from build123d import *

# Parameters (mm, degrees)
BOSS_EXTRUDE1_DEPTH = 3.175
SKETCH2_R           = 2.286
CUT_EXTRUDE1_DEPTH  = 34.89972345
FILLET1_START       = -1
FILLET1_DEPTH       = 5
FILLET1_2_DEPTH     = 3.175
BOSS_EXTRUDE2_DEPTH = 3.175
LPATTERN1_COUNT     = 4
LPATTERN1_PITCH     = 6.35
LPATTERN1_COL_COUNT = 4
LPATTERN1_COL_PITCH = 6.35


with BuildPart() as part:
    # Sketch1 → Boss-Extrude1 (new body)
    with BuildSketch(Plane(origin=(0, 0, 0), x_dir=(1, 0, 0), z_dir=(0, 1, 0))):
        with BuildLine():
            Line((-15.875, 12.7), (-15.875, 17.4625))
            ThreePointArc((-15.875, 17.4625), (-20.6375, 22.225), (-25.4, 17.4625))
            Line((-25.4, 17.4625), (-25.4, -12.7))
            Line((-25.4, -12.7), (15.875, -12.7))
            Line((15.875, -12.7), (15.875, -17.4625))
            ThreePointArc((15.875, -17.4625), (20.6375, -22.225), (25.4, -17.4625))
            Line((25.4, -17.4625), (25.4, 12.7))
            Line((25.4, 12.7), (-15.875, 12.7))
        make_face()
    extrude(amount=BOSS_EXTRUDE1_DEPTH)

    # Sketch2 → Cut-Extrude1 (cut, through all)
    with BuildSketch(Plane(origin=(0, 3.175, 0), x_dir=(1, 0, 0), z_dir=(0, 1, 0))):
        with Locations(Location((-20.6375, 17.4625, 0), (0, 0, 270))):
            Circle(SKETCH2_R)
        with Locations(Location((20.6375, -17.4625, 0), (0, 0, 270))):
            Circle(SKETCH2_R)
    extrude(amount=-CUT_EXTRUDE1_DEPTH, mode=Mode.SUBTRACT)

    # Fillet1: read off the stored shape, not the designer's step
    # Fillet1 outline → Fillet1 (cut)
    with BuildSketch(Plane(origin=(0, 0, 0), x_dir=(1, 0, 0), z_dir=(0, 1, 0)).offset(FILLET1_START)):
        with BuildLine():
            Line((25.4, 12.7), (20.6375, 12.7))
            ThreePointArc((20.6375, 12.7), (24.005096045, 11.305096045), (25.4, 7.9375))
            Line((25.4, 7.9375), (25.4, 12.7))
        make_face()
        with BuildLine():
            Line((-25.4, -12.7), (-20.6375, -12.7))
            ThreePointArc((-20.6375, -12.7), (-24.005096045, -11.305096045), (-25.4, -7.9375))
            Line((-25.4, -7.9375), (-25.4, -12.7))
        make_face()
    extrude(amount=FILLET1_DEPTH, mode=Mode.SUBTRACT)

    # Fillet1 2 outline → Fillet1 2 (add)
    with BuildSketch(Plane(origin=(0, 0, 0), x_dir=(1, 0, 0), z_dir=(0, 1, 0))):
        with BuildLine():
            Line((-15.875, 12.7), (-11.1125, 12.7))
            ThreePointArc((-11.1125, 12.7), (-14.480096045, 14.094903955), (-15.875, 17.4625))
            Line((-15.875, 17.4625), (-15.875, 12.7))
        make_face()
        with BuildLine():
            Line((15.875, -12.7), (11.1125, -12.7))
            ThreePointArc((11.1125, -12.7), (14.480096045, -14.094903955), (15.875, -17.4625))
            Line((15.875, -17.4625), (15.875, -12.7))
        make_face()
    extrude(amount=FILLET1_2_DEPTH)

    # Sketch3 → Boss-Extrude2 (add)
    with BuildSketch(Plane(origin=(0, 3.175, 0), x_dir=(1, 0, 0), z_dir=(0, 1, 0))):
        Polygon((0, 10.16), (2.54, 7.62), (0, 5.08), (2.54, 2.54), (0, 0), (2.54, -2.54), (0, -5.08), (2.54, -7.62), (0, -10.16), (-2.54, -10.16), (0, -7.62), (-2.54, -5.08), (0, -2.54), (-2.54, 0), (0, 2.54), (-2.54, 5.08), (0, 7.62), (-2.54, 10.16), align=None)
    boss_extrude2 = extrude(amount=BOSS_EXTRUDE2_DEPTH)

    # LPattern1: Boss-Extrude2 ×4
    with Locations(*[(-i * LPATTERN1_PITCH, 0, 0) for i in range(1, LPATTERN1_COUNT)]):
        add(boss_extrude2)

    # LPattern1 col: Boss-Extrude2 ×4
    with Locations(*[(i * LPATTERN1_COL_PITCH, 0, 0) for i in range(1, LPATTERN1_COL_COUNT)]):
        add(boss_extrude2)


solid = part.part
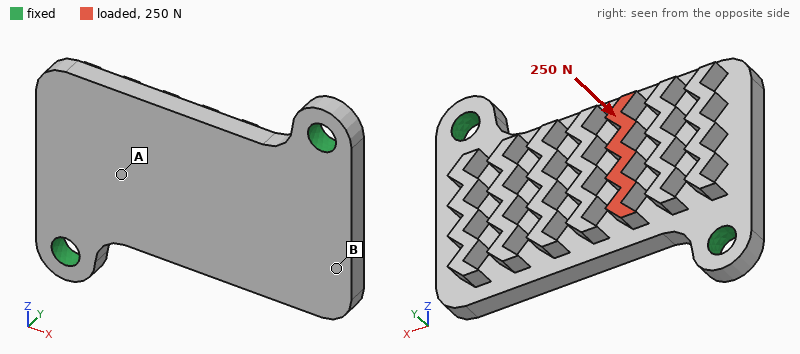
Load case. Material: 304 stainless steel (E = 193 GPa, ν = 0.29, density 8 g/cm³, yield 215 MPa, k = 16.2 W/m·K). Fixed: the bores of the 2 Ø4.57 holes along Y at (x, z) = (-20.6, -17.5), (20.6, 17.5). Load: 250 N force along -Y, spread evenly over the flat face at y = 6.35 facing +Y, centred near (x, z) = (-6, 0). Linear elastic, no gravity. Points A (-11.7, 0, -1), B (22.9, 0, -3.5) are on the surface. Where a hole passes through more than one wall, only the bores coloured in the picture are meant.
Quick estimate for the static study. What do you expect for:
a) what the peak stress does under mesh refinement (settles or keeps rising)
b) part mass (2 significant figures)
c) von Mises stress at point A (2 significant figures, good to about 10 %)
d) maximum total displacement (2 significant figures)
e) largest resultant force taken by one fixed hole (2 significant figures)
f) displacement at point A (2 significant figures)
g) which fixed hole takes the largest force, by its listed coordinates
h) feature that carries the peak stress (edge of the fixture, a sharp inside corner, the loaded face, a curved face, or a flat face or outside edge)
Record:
keeps rising
45 g
20 MPa
31 µm
160 N
17 µm
(-20.6, -17.5)
edge of the fixture
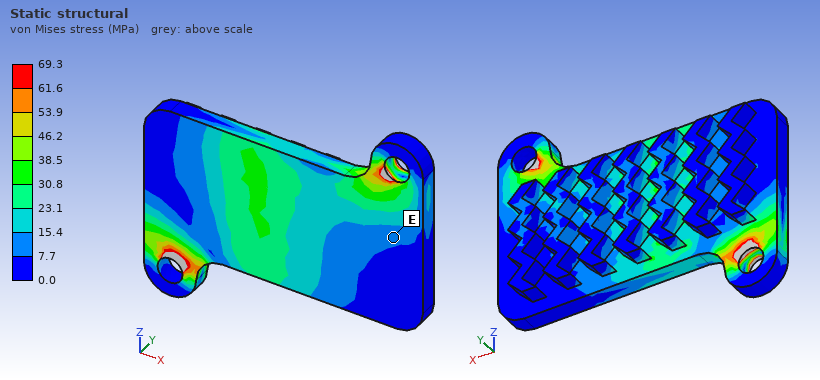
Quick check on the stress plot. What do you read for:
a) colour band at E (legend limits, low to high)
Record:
7.7 to 15.4 MPa
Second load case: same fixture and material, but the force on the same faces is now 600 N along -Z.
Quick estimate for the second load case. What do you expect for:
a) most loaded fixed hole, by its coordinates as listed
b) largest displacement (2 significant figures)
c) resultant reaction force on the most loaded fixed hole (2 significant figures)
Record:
(-20.6, -17.5)
41 µm
410 N
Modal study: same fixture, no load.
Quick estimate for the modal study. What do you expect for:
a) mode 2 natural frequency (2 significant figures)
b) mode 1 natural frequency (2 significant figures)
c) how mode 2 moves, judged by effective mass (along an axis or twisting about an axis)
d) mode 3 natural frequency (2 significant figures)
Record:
3600 Hz
3000 Hz
along Y
8400 Hz
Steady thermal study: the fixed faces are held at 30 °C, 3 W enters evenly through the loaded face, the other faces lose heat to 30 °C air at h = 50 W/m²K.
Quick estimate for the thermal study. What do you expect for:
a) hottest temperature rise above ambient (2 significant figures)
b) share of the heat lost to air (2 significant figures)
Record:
31 K
72 %
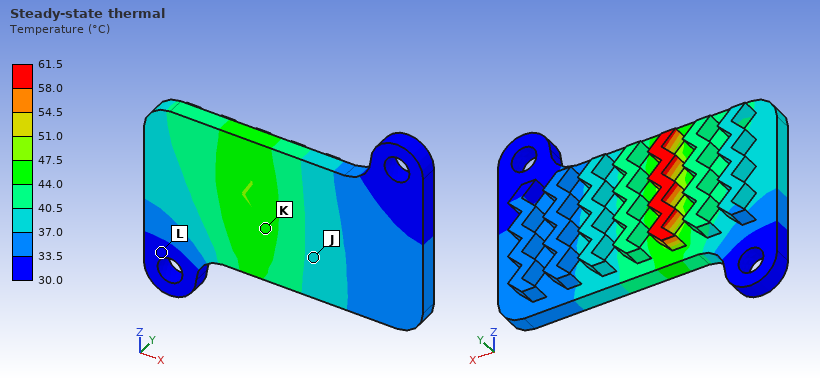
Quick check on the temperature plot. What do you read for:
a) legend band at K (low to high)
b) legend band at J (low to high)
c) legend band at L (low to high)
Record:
44.0 to 47.5 °C
37.0 to 40.5 °C
30.0 to 33.5 °C
